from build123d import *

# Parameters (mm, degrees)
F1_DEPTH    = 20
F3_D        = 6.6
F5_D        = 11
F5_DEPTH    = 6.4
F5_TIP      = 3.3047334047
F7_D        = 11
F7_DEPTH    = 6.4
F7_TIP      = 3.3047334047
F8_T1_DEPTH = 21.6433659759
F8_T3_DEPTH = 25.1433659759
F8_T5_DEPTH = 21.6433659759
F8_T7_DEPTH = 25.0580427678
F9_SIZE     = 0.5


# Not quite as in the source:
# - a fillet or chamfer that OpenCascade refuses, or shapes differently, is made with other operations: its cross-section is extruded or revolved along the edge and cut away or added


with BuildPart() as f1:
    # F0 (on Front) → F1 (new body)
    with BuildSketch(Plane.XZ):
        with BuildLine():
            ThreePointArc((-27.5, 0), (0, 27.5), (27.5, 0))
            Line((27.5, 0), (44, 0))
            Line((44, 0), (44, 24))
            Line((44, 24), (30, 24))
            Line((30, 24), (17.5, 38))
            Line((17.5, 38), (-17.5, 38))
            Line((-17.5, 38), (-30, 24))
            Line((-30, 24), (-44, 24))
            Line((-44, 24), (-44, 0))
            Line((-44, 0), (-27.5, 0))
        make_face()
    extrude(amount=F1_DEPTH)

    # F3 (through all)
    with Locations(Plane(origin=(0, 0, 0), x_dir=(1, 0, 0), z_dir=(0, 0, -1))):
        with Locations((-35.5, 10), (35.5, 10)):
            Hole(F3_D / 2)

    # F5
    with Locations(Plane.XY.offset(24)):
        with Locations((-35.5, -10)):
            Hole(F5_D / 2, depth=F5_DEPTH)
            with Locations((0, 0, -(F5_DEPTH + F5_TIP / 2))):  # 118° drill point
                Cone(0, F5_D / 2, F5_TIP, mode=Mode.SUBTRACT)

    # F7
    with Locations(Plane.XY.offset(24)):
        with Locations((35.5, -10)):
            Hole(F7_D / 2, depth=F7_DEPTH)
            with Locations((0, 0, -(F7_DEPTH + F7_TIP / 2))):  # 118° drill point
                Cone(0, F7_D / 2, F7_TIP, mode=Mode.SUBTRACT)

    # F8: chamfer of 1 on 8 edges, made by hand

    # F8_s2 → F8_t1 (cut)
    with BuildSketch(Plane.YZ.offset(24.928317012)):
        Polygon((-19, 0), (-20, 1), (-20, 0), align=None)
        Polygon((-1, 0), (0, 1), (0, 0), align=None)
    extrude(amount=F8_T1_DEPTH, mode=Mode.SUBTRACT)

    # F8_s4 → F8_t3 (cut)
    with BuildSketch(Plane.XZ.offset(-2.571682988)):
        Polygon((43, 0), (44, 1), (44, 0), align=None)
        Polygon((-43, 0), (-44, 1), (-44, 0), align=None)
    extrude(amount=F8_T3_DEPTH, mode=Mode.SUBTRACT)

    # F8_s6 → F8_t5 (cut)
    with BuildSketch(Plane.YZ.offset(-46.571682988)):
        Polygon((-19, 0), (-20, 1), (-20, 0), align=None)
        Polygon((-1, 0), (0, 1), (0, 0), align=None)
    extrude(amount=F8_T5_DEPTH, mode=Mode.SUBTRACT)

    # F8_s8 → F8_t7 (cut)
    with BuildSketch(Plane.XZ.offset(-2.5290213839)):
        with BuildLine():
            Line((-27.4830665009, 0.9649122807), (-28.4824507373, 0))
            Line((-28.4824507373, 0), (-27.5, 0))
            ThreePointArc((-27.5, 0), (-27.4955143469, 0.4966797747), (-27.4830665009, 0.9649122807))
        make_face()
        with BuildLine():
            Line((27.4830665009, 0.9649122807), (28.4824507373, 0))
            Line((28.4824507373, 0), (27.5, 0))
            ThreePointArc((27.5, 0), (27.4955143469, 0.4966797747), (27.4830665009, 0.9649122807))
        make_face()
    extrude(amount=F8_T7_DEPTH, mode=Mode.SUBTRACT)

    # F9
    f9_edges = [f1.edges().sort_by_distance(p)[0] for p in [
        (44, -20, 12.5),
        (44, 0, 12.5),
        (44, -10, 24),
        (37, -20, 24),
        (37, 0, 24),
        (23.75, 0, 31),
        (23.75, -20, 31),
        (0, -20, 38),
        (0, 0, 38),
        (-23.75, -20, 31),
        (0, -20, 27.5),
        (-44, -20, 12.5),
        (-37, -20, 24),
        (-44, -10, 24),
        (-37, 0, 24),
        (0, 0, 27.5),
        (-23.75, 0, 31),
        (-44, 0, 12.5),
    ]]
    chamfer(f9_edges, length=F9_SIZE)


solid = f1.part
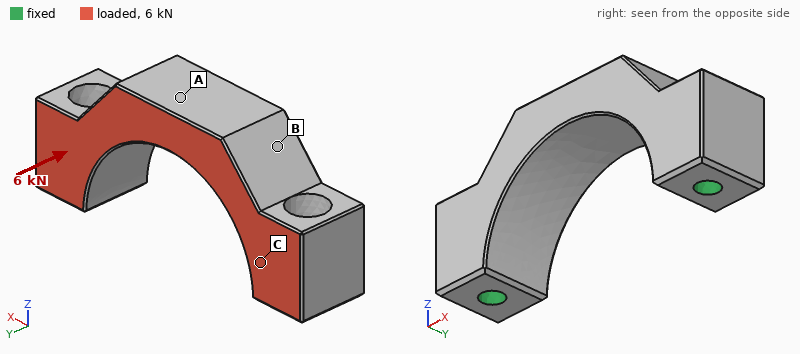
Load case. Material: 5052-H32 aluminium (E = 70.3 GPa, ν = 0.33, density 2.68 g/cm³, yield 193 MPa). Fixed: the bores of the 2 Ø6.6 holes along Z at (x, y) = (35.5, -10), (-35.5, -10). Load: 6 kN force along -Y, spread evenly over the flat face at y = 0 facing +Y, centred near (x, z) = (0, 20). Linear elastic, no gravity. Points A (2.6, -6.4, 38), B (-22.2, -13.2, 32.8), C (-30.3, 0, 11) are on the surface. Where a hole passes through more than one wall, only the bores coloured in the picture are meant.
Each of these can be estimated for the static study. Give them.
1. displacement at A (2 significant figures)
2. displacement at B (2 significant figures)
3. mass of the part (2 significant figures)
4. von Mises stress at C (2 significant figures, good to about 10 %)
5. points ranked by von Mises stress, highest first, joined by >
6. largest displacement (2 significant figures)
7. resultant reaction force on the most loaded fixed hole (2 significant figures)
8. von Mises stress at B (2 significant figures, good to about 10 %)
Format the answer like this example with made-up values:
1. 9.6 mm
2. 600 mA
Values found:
1. 40 µm
2. 28 µm
3. 78 g
4. 32 MPa
5. C > B > A
6. 42 µm
7. 3.0 kN
8. 17 MPa
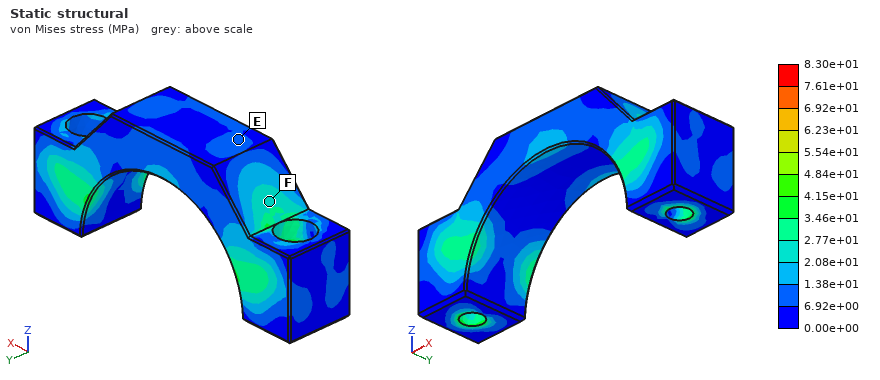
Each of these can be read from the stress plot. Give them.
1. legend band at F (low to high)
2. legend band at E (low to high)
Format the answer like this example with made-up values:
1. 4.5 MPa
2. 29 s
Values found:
1. 2.08e+01 to 2.77e+01 MPa
2. 6.92e+00 to 1.38e+01 MPa
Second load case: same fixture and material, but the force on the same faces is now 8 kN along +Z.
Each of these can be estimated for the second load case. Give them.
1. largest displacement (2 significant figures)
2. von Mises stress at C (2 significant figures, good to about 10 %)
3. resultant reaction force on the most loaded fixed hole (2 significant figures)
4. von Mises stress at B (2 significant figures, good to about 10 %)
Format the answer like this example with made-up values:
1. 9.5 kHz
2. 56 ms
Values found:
1. 44 µm
2. 33 MPa
3. 4.2 kN
4. 16 MPa
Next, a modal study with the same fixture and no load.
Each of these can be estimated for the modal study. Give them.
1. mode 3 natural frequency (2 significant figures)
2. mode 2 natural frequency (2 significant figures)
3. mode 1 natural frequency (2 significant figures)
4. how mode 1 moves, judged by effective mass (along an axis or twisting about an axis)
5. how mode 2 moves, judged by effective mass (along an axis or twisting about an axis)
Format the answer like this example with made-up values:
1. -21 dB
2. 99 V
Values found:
1. 18 kHz
2. 16 kHz
3. 7900 Hz
4. along Y
5. along X
